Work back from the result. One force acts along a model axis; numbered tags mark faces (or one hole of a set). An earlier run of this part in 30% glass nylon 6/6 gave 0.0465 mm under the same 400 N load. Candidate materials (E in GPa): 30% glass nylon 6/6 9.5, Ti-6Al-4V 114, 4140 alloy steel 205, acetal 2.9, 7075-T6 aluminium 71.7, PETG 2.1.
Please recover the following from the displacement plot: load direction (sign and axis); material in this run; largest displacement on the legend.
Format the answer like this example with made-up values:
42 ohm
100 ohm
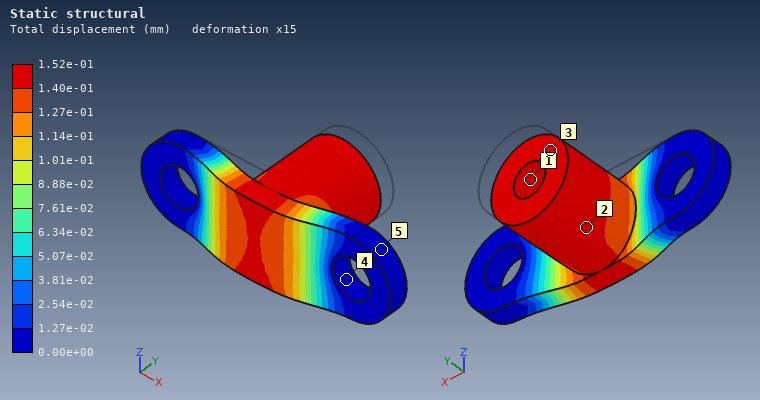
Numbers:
-Y
acetal
1.52e-01 mm
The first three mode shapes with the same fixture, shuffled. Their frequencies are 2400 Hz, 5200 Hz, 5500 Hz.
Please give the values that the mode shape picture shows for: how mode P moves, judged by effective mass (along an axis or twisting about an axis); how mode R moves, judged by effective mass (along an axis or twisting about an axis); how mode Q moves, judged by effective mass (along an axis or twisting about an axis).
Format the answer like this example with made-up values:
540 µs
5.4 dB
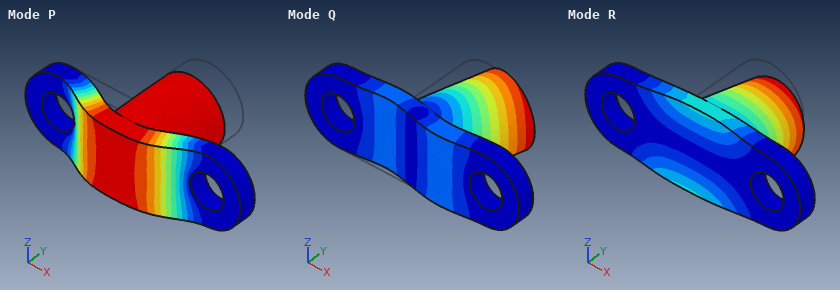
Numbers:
along Y
along Z
along X
